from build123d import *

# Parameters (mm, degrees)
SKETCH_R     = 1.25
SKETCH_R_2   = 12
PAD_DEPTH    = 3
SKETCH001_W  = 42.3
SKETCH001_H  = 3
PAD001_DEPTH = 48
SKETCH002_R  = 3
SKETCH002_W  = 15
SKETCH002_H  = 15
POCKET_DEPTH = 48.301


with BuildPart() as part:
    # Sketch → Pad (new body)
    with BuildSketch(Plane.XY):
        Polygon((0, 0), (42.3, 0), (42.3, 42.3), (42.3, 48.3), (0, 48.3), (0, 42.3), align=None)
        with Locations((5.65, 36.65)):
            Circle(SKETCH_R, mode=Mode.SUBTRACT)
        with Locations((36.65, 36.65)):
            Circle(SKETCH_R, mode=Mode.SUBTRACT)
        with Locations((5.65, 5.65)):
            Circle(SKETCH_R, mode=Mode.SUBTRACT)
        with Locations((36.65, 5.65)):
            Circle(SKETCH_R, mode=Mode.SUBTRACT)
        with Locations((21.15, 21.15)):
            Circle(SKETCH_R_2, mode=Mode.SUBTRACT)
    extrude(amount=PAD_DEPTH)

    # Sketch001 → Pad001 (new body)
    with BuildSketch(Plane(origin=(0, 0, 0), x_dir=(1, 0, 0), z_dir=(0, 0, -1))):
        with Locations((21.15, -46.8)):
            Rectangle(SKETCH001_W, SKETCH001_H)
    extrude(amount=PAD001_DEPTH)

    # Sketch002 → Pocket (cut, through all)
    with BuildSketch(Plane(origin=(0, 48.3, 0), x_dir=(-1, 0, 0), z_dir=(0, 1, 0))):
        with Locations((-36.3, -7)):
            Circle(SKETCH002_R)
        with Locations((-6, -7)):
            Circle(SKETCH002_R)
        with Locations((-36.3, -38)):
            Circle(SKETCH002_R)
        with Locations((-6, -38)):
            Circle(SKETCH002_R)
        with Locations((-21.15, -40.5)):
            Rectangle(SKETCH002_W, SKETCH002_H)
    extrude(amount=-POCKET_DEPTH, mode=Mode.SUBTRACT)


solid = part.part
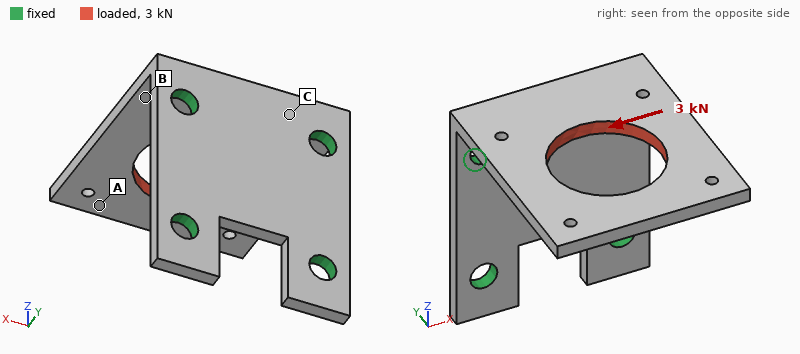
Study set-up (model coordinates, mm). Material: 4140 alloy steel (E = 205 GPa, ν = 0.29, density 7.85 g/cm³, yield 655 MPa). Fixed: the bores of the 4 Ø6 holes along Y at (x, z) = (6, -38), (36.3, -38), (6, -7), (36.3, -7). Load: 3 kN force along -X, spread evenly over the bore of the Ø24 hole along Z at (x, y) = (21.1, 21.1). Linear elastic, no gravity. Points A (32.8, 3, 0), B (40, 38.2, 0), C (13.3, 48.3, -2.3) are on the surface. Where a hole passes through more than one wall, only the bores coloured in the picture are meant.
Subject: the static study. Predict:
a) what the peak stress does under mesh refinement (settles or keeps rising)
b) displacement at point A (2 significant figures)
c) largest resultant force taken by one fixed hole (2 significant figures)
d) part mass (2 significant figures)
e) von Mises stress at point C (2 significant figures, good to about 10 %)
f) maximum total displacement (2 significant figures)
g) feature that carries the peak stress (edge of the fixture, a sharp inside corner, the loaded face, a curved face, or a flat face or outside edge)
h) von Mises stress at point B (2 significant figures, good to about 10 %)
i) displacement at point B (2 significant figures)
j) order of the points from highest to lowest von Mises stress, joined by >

keeps rising
0.14 mm
2.9 kN
77 g
86 MPa
0.16 mm
edge of the fixture
170 MPa
0.054 mm
B > C > A
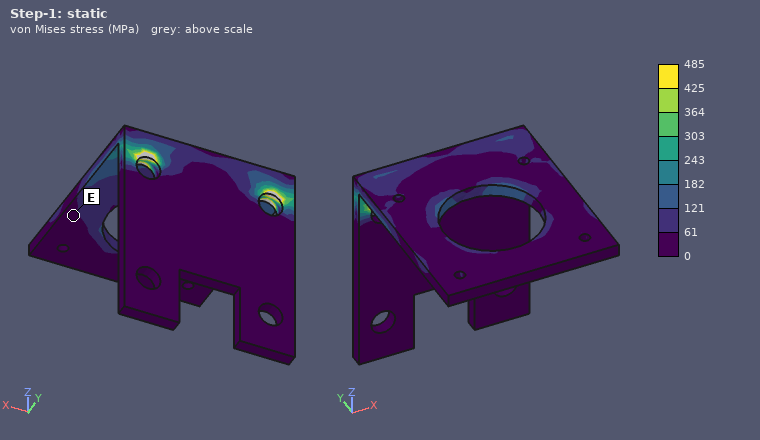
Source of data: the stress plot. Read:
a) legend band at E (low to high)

0 to 61 MPa
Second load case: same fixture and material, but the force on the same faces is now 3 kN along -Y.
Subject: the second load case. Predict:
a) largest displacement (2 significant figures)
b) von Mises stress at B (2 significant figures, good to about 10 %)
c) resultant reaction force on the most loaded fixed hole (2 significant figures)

0.19 mm
55 MPa
1.5 kN
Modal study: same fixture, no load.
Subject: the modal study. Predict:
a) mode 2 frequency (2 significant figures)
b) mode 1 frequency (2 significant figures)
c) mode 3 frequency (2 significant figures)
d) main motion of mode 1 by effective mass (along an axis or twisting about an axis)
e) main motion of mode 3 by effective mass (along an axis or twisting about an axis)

2400 Hz
930 Hz
4800 Hz
along Z
along X
